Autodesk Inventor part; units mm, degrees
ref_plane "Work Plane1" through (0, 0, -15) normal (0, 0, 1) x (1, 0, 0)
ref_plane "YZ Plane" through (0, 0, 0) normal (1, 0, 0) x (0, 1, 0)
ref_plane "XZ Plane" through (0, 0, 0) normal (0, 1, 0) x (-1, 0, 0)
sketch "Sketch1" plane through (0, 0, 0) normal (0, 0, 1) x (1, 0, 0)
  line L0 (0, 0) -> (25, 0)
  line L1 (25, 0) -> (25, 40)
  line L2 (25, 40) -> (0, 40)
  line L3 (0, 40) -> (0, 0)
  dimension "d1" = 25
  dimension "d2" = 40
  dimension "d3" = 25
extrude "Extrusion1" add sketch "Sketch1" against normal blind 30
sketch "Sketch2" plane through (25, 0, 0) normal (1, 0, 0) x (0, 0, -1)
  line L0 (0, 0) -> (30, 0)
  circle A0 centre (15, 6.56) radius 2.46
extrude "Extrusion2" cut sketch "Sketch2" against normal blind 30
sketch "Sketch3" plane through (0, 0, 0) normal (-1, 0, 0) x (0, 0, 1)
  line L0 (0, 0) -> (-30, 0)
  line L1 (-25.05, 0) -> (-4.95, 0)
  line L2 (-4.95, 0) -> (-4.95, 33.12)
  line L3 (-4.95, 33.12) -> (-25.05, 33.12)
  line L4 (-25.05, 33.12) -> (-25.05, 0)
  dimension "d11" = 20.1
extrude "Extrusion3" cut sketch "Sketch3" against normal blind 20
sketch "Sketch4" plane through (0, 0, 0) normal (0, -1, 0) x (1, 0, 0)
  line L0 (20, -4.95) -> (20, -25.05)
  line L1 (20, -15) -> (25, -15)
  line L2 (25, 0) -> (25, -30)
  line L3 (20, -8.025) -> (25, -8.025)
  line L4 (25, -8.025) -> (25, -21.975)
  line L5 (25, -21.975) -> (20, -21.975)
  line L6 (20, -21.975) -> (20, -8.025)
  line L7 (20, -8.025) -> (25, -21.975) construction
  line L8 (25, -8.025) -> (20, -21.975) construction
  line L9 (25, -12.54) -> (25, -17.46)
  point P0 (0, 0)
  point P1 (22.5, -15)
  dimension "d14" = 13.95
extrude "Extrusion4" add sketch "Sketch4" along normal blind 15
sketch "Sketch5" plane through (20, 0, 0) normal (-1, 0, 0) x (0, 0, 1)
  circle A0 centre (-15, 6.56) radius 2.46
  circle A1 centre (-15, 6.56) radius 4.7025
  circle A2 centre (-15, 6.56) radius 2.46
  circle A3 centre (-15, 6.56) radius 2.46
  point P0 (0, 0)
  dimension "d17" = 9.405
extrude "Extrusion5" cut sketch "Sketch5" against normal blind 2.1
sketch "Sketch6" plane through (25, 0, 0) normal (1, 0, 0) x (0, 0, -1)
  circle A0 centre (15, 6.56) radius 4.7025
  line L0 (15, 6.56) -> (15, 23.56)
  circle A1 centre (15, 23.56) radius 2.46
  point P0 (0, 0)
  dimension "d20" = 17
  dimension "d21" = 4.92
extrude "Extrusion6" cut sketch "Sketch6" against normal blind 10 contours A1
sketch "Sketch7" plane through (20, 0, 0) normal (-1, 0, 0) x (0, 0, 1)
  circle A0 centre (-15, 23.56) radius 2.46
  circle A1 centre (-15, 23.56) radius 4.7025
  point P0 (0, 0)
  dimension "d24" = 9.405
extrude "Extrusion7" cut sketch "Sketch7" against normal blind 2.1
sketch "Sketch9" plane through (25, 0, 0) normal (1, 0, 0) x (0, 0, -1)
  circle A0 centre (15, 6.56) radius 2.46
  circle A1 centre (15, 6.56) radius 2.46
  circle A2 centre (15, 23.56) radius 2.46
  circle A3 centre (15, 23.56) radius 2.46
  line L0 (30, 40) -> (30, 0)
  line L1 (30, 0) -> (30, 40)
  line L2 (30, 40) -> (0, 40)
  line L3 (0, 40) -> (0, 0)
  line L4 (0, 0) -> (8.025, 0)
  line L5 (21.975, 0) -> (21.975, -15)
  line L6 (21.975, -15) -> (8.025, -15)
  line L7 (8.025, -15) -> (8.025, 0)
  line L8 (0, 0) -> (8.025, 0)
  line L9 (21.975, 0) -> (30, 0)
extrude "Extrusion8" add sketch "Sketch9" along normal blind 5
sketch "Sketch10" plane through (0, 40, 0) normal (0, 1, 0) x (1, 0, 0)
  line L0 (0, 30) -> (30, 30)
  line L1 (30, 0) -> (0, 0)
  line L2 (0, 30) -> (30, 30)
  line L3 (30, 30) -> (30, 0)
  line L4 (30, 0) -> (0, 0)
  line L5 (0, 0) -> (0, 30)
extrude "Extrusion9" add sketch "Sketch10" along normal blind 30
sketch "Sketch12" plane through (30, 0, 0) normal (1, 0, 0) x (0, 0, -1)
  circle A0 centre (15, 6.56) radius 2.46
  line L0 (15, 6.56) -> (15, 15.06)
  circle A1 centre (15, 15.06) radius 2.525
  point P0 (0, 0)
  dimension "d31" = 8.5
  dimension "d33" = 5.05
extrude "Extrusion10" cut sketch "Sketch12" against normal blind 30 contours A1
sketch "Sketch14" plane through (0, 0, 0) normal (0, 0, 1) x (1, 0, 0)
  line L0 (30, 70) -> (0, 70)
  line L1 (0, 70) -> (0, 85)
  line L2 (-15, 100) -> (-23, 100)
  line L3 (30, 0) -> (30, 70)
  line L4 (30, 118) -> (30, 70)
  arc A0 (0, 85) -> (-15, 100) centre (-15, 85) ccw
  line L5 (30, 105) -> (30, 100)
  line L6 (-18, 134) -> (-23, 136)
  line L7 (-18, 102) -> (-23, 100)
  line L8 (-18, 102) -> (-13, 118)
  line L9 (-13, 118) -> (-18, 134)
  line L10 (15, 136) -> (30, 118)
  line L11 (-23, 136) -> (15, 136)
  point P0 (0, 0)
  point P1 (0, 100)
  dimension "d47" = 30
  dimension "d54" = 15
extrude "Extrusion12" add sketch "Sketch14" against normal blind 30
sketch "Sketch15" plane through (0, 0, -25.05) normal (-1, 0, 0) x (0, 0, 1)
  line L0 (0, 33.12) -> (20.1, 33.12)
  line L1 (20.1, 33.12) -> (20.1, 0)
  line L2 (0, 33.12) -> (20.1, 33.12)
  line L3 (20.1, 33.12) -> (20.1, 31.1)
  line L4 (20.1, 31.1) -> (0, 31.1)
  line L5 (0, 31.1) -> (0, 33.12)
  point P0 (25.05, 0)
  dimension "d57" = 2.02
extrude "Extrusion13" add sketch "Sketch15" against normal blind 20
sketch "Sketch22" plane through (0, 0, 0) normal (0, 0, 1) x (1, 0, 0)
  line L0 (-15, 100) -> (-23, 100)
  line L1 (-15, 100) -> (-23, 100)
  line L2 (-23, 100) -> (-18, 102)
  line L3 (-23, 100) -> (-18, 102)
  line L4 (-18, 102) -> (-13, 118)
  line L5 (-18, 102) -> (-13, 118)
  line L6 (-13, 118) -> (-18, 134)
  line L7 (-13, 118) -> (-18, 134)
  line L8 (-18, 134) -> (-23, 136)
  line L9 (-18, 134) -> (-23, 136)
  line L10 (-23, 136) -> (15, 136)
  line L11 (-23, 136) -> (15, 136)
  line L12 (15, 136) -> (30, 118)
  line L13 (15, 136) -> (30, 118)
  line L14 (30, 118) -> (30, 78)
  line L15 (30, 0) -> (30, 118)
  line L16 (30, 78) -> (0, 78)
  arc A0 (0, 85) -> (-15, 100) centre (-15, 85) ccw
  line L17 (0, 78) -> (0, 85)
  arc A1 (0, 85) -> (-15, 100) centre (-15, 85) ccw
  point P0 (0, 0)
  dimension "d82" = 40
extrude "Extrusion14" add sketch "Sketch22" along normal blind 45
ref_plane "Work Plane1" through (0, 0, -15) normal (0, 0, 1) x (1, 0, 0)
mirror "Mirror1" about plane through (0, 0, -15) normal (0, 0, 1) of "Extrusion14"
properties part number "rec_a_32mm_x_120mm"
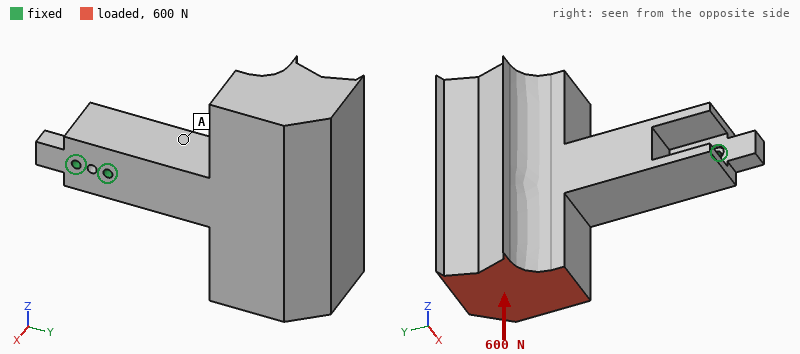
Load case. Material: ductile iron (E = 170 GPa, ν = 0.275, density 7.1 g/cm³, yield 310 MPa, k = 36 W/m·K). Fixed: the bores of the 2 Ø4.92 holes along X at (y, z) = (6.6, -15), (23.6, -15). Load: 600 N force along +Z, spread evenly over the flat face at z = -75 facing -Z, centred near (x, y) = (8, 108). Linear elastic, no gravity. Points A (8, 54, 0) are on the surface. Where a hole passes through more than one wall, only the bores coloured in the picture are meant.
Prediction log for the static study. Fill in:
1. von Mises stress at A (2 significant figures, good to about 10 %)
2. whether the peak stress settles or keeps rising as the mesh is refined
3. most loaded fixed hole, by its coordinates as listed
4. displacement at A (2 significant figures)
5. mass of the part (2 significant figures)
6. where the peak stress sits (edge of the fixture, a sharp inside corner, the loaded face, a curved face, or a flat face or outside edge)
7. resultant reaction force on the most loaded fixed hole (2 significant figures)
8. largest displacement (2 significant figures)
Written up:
7.1 MPa
keeps rising
(23.6, -15)
13 µm
2.3 kg
edge of the fixture
2.8 kN
59 µm
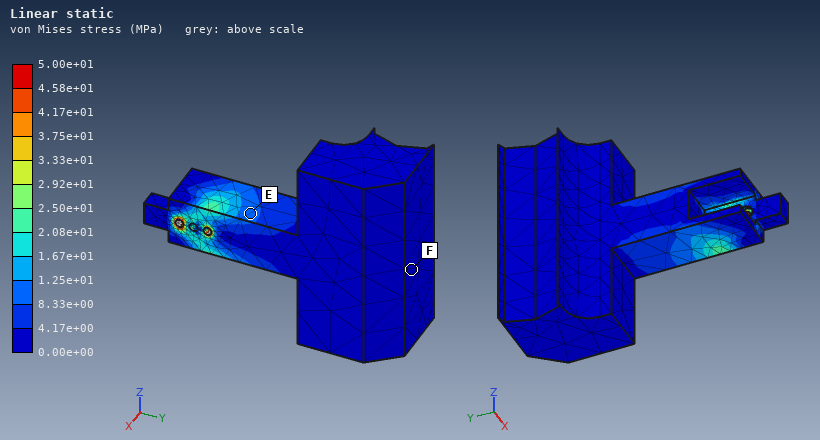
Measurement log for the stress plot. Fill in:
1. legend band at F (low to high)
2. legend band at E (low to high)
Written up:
0.00e+00 to 4.17e+00 MPa
8.33e+00 to 1.25e+01 MPa
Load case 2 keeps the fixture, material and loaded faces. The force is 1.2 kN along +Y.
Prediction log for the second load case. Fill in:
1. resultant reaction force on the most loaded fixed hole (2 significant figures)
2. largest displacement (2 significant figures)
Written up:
3.3 kN
0.10 mm
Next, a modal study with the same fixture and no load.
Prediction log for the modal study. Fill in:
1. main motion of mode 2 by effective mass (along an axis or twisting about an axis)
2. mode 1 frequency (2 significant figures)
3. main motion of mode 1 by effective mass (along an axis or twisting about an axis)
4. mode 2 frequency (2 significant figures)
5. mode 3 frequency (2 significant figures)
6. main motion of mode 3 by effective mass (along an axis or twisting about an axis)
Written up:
along Z
390 Hz
along X
420 Hz
610 Hz
twisting about Y
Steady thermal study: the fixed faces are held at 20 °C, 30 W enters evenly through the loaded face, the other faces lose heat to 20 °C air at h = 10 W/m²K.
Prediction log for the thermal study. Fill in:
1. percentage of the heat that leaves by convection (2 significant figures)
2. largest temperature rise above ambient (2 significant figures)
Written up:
50 %
65 K
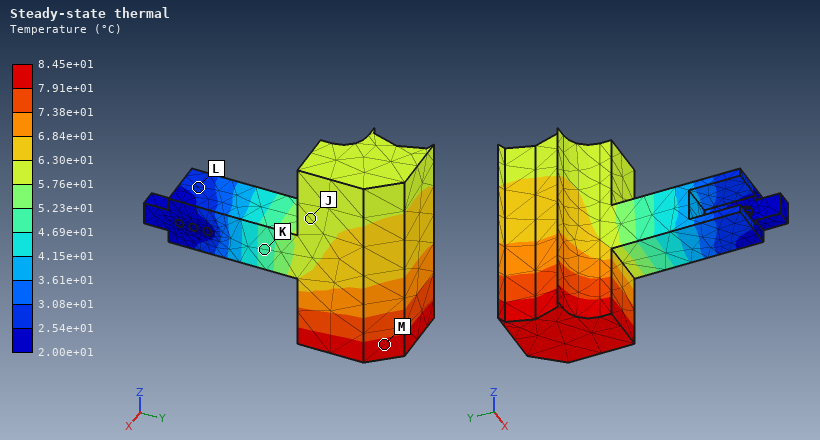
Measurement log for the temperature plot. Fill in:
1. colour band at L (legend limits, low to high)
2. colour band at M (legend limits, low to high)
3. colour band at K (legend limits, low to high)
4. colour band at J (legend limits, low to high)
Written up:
2.54e+01 to 3.08e+01 °C
7.91e+01 to 8.45e+01 °C
4.69e+01 to 5.23e+01 °C
5.76e+01 to 6.30e+01 °C
